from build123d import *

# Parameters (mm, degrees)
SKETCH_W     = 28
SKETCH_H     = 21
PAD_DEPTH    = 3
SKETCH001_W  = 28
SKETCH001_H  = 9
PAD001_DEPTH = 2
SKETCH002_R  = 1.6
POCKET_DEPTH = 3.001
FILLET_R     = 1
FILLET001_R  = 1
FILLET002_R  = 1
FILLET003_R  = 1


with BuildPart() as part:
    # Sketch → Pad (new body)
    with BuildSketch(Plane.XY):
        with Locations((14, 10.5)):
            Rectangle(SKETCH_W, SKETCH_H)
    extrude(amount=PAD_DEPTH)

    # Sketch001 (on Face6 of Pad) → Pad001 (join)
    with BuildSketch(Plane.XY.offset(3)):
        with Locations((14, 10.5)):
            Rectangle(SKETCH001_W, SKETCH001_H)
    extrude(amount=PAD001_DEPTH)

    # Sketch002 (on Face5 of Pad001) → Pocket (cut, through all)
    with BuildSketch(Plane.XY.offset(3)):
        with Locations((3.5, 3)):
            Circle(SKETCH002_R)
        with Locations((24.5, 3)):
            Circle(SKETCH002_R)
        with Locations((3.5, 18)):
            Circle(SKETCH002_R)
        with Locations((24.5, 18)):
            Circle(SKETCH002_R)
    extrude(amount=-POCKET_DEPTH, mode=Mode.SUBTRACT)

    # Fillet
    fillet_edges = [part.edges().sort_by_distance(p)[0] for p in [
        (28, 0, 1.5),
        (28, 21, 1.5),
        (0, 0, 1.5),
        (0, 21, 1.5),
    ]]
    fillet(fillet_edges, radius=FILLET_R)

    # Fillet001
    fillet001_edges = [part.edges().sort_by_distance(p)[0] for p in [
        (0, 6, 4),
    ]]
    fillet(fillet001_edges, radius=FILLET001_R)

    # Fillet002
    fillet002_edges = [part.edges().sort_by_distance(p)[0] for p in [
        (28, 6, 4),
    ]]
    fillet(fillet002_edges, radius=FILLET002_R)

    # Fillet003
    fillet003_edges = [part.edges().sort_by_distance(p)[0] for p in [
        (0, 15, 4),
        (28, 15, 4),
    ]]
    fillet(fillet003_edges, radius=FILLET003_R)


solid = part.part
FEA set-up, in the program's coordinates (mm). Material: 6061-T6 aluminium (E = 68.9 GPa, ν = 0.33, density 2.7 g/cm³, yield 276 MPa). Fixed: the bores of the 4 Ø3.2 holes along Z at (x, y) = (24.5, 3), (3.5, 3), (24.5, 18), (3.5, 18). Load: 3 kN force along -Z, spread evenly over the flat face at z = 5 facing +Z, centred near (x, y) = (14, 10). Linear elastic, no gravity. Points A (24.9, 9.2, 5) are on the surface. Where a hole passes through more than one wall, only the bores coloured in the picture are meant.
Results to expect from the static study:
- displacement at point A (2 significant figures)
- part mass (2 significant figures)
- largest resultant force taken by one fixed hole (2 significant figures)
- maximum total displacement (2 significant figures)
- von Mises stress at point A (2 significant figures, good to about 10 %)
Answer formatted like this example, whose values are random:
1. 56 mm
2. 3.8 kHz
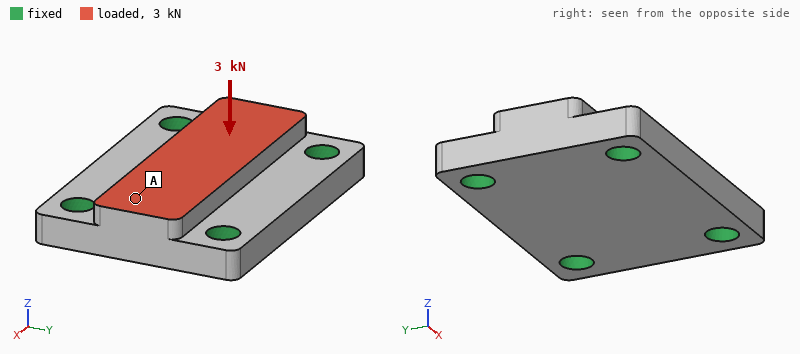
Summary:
1. 7.0 µm
2. 5.9 g
3. 810 N
4. 16 µm
5. 34 MPa
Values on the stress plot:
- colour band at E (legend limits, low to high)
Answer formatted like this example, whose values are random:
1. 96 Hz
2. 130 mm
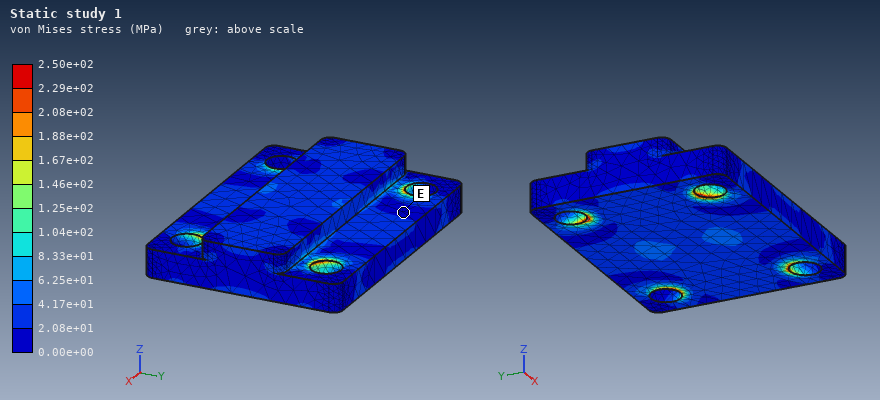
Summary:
1. 0.00e+00 to 2.08e+01 MPa
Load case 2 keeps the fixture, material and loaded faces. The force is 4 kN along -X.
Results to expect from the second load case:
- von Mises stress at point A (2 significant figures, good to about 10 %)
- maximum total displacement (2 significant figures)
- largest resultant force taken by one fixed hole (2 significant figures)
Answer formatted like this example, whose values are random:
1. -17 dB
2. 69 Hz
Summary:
1. 46 MPa
2. 14 µm
3. 1.1 kN
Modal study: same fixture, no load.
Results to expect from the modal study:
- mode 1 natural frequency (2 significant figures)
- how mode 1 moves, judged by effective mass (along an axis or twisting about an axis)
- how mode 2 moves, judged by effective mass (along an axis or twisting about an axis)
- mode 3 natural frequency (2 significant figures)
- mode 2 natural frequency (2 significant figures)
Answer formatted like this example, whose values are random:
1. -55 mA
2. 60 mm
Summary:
1. 34 kHz
2. along Z
3. twisting about X
4. 63 kHz
5. 46 kHz
